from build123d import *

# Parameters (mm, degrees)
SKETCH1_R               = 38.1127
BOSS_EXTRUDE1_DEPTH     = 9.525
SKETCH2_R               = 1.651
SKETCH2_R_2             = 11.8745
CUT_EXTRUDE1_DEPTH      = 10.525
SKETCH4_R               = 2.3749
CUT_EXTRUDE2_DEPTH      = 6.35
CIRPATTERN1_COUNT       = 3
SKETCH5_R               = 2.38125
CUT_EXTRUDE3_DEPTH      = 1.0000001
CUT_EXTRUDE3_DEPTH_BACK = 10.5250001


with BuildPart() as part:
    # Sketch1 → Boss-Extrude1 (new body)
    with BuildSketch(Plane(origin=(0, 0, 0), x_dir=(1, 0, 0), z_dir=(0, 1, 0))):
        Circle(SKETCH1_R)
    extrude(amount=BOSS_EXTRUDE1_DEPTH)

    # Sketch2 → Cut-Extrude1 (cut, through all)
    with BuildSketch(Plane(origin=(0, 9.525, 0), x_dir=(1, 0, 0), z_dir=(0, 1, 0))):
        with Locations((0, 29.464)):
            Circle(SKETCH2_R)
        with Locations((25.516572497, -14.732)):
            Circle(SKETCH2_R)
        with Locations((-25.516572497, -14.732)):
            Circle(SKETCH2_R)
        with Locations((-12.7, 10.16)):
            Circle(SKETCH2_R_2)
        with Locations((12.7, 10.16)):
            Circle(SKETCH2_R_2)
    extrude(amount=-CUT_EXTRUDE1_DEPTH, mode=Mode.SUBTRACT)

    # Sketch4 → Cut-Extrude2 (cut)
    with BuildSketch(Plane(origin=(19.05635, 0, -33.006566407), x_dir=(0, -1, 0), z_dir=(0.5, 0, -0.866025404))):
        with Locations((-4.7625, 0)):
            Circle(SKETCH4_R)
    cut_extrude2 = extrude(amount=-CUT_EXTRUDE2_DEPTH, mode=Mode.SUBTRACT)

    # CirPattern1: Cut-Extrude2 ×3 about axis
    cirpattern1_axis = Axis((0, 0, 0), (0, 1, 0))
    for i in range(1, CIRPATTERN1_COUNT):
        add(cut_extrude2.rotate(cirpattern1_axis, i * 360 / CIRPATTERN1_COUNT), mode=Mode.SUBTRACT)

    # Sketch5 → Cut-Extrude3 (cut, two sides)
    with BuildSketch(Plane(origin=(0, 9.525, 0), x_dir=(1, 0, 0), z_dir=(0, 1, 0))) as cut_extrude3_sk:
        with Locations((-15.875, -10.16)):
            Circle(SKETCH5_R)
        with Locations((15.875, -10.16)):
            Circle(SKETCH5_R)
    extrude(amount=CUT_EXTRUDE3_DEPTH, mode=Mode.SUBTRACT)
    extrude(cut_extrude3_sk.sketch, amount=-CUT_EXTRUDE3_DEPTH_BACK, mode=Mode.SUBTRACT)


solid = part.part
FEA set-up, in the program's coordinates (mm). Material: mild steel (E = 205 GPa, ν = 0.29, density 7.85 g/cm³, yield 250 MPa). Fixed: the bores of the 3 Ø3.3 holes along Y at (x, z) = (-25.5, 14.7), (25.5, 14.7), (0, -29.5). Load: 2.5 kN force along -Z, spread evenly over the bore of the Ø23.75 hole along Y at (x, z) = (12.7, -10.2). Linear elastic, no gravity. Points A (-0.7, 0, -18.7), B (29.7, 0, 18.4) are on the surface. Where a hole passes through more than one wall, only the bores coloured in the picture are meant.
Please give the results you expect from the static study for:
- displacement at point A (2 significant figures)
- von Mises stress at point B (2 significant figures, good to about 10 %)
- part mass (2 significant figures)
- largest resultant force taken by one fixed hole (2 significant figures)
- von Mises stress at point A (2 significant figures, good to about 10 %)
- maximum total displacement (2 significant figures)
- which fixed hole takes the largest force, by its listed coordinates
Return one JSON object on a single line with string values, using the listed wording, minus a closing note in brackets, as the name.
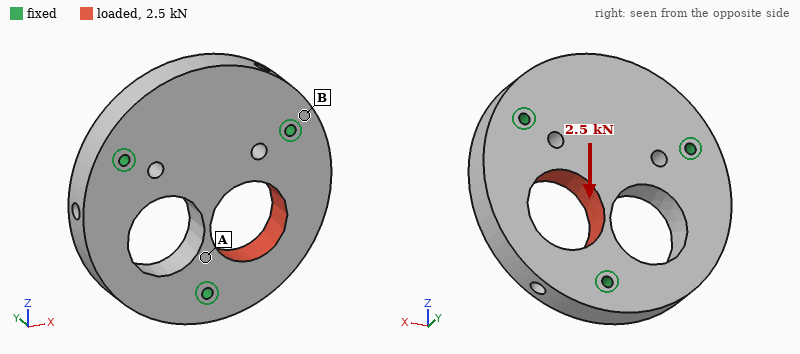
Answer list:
{"displacement at point A": "0.63 µm", "von Mises stress at point B": "3.4 MPa", "part mass": "270 g", "largest resultant force taken by one fixed hole": "1.4 kN", "von Mises stress at point A": "7.7 MPa", "maximum total displacement": "1.6 µm", "which fixed hole takes the largest force, by its listed coordinates": "(25.5, 14.7)"}
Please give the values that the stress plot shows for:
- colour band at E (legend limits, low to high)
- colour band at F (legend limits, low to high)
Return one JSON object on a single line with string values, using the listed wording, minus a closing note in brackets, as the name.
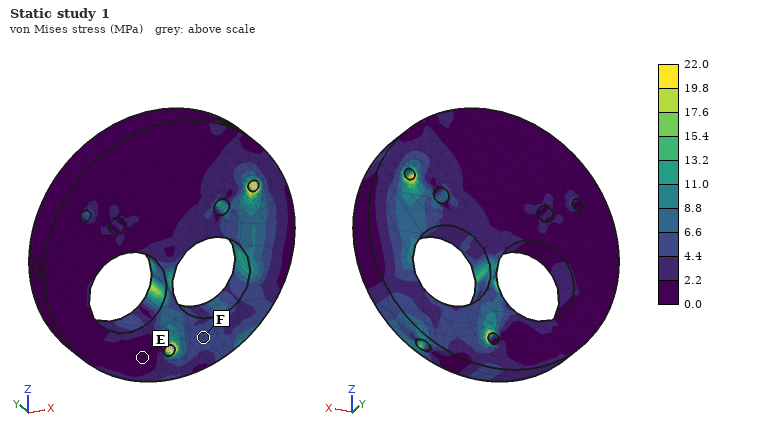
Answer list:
{"colour band at E": "0.0 to 2.2 MPa", "colour band at F": "4.4 to 6.6 MPa"}
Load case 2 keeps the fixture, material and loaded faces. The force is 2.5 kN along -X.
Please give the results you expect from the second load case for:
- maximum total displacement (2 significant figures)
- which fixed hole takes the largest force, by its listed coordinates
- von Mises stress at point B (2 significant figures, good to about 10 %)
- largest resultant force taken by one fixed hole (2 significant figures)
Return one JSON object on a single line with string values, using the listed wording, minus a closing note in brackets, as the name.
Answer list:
{"maximum total displacement": "2.4 µm", "which fixed hole takes the largest force, by its listed coordinates": "(0, -29.5)", "von Mises stress at point B": "2.7 MPa", "largest resultant force taken by one fixed hole": "1.3 kN"}
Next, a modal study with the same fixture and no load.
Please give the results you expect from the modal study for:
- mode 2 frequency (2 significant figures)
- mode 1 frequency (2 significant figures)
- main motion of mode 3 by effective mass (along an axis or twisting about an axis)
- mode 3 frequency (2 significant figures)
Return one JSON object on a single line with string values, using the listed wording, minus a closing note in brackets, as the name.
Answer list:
{"mode 2 frequency": "9000 Hz", "mode 1 frequency": "8800 Hz", "main motion of mode 3 by effective mass": "along Y", "mode 3 frequency": "10 kHz"}
